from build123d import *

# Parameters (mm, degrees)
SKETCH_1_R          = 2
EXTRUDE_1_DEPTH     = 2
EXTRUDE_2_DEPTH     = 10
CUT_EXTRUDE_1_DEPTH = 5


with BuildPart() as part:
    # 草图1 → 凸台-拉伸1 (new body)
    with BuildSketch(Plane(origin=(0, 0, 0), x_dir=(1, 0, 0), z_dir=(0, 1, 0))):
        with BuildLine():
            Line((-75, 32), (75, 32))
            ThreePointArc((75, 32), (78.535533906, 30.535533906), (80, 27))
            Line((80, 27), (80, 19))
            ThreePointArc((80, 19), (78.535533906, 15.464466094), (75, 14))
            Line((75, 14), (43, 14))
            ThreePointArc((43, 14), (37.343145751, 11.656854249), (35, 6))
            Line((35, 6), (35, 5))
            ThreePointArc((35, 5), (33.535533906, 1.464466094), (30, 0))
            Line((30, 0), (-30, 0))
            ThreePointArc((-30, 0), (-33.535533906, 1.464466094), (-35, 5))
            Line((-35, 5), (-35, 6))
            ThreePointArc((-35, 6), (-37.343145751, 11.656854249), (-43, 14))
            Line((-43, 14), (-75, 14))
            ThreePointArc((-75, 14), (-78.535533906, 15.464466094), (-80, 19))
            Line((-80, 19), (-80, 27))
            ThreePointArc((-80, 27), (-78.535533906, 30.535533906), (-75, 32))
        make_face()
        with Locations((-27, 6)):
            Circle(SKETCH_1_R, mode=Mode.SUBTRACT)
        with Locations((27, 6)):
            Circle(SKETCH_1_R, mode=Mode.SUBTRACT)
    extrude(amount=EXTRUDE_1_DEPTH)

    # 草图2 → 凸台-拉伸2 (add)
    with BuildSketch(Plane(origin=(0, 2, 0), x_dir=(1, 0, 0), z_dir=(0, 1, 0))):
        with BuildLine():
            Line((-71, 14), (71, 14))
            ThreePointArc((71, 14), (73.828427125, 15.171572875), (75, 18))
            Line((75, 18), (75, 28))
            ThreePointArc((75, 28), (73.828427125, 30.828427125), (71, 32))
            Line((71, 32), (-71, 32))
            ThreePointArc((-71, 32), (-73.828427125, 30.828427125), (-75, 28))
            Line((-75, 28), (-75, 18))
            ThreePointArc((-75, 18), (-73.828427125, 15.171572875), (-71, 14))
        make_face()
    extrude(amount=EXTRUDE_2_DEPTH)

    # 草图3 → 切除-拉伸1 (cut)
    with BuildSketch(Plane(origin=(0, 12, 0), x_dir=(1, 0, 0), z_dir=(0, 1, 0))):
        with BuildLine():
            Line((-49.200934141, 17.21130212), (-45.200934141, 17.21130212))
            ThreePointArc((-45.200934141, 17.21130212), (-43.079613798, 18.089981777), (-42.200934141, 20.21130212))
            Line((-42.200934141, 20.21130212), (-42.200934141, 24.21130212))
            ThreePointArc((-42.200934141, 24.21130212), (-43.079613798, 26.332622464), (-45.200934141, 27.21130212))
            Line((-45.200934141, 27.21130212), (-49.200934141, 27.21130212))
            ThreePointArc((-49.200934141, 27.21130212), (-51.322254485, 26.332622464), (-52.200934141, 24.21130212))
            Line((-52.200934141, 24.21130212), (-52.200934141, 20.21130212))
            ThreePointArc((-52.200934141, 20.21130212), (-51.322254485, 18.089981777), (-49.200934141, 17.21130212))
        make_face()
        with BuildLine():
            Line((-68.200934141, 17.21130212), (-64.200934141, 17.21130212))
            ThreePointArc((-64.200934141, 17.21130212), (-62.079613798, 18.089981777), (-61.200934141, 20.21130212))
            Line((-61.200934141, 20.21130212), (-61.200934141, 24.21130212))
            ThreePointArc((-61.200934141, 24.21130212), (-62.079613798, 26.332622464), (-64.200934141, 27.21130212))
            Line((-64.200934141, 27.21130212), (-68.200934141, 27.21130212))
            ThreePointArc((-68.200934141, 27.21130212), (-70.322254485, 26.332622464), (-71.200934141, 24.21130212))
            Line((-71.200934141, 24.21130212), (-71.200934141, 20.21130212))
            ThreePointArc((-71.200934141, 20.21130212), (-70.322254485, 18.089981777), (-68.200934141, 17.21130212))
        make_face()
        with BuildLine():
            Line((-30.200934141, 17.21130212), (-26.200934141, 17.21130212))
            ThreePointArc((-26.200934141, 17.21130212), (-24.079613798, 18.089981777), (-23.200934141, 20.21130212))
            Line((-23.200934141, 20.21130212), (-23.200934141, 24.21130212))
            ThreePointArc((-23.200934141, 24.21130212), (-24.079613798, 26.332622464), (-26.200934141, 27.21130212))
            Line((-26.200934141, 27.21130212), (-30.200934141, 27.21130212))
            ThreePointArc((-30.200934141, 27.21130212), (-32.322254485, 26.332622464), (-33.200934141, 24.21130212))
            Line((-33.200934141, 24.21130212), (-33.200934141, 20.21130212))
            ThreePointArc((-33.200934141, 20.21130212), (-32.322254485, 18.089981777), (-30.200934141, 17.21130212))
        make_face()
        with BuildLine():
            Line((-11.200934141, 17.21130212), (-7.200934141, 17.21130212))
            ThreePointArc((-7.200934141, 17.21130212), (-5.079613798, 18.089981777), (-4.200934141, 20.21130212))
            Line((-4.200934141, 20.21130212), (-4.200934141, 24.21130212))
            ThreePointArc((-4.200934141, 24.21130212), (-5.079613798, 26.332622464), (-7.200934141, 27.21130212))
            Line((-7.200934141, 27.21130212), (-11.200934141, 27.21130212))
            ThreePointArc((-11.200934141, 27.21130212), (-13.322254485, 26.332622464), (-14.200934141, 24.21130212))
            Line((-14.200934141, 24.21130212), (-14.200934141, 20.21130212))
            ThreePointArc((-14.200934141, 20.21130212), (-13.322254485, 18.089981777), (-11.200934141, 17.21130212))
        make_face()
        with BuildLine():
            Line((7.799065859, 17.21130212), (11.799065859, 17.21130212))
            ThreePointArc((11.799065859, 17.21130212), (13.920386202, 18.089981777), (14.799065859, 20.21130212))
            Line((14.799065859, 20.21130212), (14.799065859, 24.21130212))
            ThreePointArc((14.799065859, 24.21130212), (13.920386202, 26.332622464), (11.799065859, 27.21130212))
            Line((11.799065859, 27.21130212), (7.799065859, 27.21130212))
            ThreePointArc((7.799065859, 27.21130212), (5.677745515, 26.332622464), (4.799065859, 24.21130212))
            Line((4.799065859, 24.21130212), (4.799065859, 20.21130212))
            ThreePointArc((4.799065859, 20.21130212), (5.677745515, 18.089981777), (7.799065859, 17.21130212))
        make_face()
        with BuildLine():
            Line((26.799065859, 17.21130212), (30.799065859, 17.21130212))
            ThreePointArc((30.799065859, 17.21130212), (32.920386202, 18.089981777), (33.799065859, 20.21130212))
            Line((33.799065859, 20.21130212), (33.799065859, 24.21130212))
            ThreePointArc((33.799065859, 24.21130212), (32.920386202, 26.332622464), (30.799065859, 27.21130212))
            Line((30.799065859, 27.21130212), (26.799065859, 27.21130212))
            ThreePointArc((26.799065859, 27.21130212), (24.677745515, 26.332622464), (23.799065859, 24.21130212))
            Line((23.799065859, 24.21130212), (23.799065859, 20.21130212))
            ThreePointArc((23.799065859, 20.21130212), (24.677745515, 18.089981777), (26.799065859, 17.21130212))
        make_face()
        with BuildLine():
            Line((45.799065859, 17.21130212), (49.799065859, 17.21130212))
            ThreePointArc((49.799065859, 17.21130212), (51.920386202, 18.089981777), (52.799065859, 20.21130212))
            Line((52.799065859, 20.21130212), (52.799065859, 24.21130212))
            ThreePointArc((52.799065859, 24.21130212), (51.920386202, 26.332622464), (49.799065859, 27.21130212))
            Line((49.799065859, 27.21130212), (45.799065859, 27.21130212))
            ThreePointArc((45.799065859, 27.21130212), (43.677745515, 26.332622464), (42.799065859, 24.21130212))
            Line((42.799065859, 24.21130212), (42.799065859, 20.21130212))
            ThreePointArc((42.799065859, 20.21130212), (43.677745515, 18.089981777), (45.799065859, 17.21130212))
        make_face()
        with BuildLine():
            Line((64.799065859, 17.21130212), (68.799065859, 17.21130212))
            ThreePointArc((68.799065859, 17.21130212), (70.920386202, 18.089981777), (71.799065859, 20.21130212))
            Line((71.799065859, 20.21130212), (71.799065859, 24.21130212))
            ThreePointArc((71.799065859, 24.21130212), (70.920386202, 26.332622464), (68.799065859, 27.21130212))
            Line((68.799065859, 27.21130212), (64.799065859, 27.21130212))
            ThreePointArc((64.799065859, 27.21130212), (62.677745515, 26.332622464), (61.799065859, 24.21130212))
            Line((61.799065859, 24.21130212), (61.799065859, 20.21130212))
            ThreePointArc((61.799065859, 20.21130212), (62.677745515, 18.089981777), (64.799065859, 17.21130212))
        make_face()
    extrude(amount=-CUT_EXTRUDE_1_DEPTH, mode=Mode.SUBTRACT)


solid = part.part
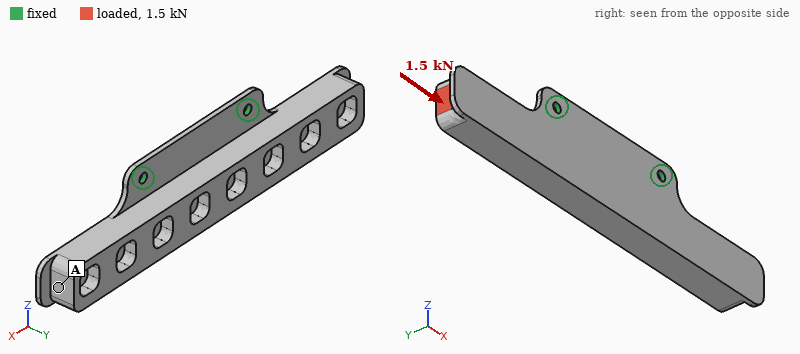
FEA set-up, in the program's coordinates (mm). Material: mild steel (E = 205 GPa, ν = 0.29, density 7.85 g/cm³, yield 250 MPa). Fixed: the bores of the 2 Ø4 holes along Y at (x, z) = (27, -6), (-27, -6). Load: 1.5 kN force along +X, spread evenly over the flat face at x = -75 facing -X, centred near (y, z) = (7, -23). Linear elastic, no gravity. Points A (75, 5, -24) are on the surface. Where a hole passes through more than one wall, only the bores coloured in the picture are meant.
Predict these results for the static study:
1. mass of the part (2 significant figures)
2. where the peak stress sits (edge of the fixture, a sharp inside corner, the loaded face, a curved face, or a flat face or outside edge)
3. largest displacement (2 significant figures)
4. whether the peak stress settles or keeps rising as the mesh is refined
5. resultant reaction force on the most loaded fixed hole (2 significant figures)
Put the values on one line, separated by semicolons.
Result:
240 g; edge of the fixture; 34 µm; keeps rising; 910 N
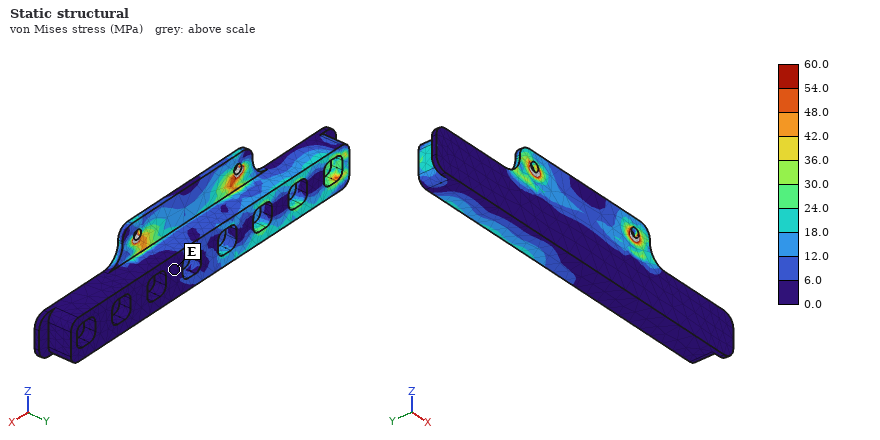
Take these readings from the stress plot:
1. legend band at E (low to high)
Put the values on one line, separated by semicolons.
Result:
0.0 to 6.0 MPa
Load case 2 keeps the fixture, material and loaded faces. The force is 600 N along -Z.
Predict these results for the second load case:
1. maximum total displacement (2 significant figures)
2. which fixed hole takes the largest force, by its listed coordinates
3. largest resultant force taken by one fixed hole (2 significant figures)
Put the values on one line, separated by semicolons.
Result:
0.15 mm; (-27, -6); 1.2 kN
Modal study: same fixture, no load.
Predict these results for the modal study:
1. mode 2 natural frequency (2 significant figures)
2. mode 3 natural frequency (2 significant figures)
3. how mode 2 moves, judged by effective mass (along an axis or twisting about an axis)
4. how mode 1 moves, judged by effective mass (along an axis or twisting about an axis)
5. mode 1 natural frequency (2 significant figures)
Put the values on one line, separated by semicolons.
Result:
1300 Hz; 2400 Hz; twisting about Z; along Y; 630 Hz
